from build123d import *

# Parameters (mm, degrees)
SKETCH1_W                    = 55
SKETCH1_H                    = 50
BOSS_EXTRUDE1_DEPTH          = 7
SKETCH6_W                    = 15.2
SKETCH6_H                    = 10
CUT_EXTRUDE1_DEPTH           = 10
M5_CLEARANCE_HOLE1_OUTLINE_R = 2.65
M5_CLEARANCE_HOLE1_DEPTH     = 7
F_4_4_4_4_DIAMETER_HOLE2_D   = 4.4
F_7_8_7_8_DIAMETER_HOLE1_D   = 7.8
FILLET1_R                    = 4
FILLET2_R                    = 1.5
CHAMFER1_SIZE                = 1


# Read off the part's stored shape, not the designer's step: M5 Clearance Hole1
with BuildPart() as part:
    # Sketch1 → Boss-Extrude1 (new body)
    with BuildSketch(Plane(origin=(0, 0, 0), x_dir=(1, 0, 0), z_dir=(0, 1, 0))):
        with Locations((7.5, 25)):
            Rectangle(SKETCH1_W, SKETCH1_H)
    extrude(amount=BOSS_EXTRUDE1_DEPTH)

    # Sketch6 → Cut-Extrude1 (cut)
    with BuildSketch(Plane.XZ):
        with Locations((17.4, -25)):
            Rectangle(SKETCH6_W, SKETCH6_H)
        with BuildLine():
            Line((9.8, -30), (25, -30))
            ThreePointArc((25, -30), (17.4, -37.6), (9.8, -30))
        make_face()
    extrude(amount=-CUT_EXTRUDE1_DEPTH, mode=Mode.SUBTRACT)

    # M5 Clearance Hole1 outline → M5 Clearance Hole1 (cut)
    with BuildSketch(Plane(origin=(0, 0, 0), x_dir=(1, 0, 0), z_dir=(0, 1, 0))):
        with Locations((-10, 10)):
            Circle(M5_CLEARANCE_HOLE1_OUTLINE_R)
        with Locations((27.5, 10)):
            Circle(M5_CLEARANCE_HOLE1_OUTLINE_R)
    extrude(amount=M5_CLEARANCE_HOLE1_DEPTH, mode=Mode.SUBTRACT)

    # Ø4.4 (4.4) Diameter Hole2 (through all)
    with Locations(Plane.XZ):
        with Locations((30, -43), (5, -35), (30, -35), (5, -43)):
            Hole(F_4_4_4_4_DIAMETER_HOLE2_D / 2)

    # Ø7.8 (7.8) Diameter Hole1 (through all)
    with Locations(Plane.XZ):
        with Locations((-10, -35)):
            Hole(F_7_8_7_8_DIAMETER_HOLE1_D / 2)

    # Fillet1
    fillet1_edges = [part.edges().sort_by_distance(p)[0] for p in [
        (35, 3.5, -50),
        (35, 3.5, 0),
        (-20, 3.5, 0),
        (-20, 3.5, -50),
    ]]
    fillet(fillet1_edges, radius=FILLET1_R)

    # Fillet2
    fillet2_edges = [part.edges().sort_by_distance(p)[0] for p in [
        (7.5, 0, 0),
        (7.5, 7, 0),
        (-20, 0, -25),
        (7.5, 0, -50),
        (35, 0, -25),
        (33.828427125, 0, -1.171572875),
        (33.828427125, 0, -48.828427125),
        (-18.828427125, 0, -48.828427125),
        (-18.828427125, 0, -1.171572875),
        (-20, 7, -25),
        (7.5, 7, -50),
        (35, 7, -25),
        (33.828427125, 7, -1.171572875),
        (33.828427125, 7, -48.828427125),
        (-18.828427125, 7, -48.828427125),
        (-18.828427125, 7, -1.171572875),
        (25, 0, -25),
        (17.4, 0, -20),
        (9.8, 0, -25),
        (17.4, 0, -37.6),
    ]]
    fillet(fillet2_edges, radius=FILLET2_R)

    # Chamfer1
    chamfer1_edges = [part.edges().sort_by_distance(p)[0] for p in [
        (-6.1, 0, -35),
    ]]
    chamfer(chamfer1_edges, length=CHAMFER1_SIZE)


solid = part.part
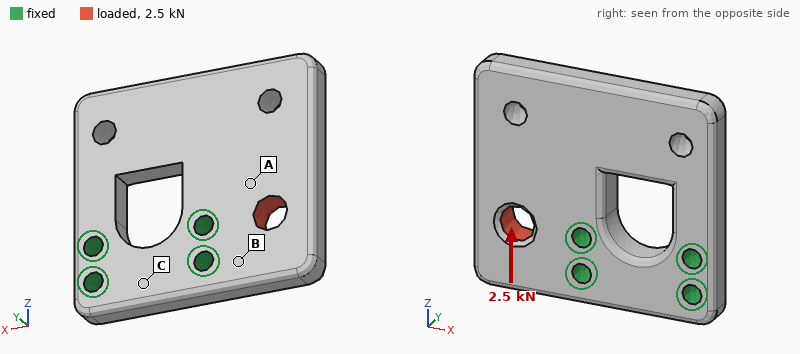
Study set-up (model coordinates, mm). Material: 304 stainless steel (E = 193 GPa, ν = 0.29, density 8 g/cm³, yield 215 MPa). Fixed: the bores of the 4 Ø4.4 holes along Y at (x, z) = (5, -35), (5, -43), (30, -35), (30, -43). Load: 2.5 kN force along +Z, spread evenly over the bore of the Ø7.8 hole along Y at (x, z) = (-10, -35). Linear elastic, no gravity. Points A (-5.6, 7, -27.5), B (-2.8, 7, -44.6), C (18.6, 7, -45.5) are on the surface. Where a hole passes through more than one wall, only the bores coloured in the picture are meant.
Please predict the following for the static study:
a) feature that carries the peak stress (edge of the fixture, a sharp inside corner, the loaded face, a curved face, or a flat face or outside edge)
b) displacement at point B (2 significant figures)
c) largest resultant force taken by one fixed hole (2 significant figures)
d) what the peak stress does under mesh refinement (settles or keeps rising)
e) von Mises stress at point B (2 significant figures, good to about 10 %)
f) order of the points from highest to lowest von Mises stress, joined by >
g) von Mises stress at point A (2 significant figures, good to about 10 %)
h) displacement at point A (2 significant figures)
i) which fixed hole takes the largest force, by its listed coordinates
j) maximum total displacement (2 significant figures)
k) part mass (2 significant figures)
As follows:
edge of the fixture
2.2 µm
2.4 kN
keeps rising
23 MPa
B > A > C
16 MPa
4.1 µm
(5, -35)
9.1 µm
130 g
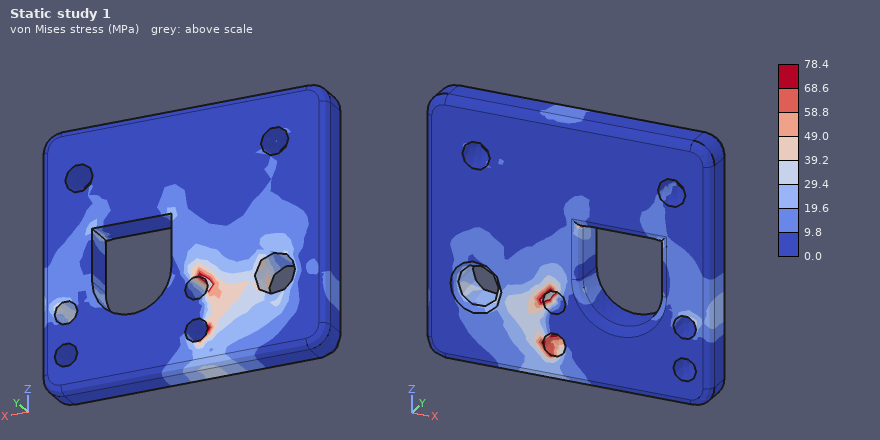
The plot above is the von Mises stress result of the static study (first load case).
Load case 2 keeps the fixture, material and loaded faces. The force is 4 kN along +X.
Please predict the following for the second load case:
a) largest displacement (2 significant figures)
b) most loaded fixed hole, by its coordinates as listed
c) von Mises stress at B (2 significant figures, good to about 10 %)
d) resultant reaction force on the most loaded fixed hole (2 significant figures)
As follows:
5.6 µm
(5, -35)
24 MPa
2.7 kN
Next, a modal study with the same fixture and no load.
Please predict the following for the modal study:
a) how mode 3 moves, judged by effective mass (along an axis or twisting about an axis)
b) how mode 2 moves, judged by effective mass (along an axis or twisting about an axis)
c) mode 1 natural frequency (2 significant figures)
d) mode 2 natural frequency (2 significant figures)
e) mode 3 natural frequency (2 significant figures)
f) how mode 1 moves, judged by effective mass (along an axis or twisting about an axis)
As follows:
along X
twisting about Z
3400 Hz
5700 Hz
8600 Hz
along Y
